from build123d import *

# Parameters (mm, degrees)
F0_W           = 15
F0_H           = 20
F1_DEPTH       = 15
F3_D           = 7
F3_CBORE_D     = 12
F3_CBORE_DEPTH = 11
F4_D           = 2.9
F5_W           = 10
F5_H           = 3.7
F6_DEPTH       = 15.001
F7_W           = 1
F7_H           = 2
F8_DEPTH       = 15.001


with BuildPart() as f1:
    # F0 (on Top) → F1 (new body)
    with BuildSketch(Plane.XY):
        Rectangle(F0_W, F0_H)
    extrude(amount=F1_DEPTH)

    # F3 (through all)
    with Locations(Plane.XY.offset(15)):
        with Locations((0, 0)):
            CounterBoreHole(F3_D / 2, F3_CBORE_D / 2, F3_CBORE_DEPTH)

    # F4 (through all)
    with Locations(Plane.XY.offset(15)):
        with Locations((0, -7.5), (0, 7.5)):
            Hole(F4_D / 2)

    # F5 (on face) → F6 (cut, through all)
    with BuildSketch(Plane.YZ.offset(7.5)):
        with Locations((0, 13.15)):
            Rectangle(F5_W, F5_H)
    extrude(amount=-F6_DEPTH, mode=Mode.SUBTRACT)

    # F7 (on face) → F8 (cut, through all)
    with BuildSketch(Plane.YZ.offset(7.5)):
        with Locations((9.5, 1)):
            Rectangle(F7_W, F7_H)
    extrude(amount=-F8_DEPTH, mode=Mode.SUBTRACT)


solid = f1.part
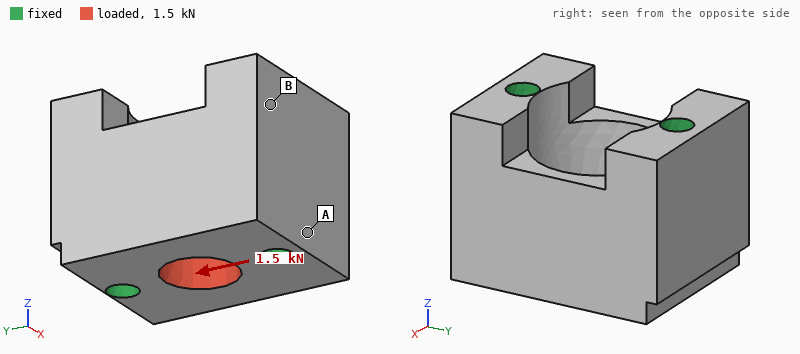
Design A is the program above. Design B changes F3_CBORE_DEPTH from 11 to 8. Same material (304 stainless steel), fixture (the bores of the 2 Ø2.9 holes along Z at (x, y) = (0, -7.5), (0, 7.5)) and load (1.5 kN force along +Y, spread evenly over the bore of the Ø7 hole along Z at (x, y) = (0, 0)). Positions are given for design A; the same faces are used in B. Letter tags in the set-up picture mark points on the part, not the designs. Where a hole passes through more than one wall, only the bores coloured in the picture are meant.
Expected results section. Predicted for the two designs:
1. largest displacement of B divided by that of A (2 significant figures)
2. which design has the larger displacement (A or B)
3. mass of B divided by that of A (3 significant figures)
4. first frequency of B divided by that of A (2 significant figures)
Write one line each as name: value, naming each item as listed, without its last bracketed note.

largest displacement of B divided by that of A: 0.64
which design has the larger displacement: A
mass of B divided by that of A: 1.08
first frequency of B divided by that of A: 1.1
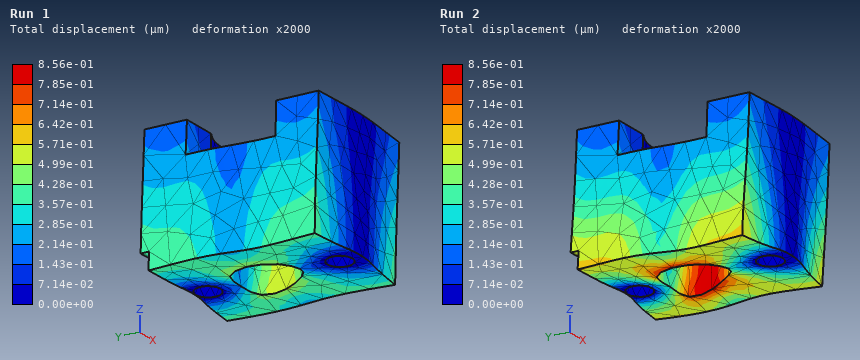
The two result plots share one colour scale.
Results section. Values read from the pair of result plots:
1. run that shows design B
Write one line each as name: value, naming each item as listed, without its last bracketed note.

run that shows design B: Run 1
